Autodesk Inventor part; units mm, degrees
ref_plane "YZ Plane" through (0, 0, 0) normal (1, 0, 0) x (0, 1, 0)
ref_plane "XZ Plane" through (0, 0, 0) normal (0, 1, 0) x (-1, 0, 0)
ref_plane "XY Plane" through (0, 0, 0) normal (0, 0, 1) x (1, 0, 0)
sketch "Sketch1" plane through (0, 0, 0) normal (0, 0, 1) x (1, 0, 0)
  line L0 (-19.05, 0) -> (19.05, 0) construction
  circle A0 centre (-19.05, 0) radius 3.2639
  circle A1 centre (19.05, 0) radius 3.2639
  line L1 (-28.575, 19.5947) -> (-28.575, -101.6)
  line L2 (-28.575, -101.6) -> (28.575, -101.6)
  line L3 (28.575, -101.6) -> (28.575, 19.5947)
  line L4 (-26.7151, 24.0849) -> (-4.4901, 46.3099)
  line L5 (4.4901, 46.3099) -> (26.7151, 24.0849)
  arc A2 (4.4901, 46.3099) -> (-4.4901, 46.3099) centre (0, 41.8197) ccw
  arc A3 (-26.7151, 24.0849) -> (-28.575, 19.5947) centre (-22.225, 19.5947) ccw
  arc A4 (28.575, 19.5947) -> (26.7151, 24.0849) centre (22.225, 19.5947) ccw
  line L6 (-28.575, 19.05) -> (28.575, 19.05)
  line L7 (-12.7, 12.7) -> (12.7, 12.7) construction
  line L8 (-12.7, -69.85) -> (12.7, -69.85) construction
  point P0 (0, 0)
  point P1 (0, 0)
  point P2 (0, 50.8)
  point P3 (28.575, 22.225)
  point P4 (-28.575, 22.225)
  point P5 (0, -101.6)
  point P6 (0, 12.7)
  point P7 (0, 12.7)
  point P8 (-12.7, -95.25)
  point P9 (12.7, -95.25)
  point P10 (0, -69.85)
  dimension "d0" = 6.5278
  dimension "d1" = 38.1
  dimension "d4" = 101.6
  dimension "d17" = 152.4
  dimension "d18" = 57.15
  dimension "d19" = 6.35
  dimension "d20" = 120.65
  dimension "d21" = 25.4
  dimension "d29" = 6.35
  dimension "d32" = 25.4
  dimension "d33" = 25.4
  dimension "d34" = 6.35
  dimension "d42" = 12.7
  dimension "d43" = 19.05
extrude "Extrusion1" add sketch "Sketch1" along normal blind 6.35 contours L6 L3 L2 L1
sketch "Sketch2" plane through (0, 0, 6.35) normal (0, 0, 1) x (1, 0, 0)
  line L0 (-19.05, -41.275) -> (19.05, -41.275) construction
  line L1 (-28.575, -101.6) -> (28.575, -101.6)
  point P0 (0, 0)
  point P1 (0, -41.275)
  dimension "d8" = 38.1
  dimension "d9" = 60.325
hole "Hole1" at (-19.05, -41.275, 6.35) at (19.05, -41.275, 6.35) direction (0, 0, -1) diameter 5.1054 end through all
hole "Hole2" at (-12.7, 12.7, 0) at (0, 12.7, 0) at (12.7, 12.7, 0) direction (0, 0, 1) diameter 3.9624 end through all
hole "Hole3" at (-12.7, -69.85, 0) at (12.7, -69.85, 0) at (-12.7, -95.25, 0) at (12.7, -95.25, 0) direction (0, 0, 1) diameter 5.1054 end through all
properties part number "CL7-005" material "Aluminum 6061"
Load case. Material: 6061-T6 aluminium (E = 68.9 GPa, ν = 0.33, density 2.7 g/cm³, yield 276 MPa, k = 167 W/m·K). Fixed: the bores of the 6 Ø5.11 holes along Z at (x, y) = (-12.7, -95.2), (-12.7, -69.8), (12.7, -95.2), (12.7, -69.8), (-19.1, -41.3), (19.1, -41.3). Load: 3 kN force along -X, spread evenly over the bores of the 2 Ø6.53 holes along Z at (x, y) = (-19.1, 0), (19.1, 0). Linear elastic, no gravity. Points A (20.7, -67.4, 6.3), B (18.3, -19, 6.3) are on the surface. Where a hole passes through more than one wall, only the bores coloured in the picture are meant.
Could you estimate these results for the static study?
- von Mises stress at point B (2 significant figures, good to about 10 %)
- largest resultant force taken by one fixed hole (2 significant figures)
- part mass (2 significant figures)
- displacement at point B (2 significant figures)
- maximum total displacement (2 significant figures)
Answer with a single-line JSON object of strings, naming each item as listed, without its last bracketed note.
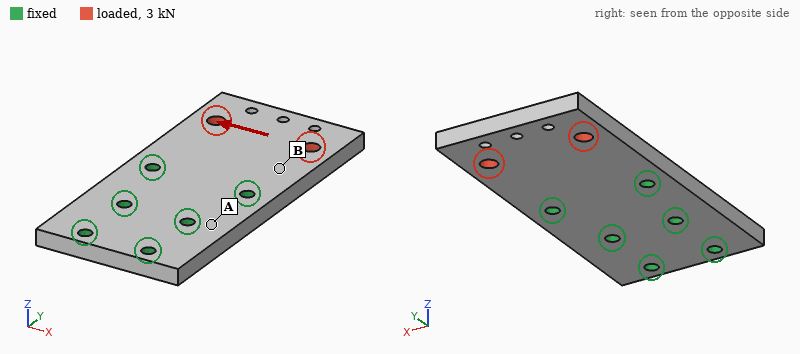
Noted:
{"von Mises stress at point B": "17 MPa", "largest resultant force taken by one fixed hole": "3.1 kN", "part mass": "110 g", "displacement at point B": "15 µm", "maximum total displacement": "39 µm"}
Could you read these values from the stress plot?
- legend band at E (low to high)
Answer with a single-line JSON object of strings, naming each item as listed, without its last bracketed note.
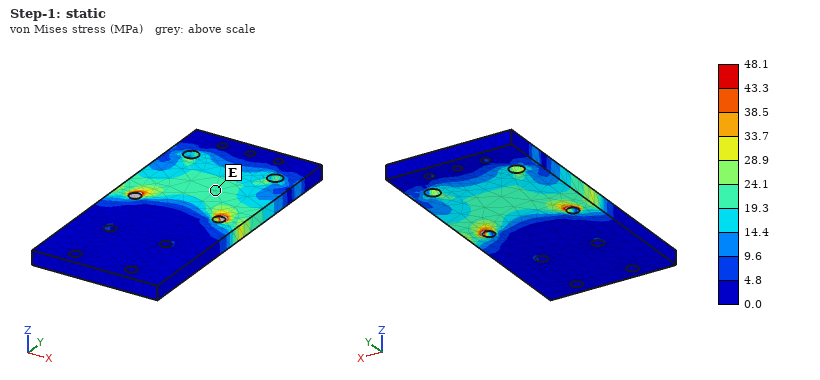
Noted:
{"legend band at E": "19.3 to 24.1 MPa"}
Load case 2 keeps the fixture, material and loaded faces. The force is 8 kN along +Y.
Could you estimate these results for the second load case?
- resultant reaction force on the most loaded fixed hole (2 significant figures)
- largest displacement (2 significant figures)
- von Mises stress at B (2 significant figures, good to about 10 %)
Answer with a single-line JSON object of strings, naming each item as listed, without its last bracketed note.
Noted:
{"resultant reaction force on the most loaded fixed hole": "3.3 kN", "largest displacement": "19 µm", "von Mises stress at B": "25 MPa"}
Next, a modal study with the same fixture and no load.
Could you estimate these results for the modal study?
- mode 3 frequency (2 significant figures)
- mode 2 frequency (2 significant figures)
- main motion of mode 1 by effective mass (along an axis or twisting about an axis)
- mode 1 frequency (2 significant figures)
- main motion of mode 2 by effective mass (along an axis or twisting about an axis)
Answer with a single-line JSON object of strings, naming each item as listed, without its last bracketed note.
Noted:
{"mode 3 frequency": "8100 Hz", "mode 2 frequency": "3500 Hz", "main motion of mode 1 by effective mass": "along Z", "mode 1 frequency": "1400 Hz", "main motion of mode 2 by effective mass": "twisting about Y"}
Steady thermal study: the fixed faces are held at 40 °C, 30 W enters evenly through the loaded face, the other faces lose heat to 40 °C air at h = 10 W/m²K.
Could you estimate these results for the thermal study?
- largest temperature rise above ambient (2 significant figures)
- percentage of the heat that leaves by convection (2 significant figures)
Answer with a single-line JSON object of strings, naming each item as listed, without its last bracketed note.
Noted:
{"largest temperature rise above ambient": "24 K", "percentage of the heat that leaves by convection": "4.0 %"}
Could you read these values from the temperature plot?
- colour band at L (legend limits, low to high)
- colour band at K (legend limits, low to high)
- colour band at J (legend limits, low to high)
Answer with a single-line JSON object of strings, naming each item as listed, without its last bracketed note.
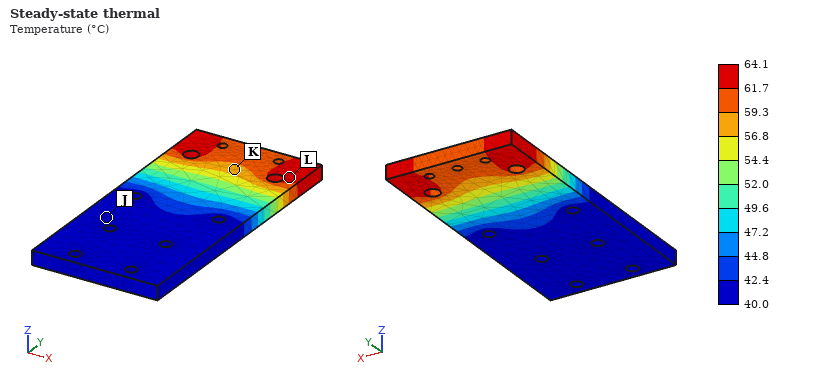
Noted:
{"colour band at L": "61.7 to 64.1 °C", "colour band at K": "56.8 to 59.3 °C", "colour band at J": "40.0 to 42.4 °C"}
